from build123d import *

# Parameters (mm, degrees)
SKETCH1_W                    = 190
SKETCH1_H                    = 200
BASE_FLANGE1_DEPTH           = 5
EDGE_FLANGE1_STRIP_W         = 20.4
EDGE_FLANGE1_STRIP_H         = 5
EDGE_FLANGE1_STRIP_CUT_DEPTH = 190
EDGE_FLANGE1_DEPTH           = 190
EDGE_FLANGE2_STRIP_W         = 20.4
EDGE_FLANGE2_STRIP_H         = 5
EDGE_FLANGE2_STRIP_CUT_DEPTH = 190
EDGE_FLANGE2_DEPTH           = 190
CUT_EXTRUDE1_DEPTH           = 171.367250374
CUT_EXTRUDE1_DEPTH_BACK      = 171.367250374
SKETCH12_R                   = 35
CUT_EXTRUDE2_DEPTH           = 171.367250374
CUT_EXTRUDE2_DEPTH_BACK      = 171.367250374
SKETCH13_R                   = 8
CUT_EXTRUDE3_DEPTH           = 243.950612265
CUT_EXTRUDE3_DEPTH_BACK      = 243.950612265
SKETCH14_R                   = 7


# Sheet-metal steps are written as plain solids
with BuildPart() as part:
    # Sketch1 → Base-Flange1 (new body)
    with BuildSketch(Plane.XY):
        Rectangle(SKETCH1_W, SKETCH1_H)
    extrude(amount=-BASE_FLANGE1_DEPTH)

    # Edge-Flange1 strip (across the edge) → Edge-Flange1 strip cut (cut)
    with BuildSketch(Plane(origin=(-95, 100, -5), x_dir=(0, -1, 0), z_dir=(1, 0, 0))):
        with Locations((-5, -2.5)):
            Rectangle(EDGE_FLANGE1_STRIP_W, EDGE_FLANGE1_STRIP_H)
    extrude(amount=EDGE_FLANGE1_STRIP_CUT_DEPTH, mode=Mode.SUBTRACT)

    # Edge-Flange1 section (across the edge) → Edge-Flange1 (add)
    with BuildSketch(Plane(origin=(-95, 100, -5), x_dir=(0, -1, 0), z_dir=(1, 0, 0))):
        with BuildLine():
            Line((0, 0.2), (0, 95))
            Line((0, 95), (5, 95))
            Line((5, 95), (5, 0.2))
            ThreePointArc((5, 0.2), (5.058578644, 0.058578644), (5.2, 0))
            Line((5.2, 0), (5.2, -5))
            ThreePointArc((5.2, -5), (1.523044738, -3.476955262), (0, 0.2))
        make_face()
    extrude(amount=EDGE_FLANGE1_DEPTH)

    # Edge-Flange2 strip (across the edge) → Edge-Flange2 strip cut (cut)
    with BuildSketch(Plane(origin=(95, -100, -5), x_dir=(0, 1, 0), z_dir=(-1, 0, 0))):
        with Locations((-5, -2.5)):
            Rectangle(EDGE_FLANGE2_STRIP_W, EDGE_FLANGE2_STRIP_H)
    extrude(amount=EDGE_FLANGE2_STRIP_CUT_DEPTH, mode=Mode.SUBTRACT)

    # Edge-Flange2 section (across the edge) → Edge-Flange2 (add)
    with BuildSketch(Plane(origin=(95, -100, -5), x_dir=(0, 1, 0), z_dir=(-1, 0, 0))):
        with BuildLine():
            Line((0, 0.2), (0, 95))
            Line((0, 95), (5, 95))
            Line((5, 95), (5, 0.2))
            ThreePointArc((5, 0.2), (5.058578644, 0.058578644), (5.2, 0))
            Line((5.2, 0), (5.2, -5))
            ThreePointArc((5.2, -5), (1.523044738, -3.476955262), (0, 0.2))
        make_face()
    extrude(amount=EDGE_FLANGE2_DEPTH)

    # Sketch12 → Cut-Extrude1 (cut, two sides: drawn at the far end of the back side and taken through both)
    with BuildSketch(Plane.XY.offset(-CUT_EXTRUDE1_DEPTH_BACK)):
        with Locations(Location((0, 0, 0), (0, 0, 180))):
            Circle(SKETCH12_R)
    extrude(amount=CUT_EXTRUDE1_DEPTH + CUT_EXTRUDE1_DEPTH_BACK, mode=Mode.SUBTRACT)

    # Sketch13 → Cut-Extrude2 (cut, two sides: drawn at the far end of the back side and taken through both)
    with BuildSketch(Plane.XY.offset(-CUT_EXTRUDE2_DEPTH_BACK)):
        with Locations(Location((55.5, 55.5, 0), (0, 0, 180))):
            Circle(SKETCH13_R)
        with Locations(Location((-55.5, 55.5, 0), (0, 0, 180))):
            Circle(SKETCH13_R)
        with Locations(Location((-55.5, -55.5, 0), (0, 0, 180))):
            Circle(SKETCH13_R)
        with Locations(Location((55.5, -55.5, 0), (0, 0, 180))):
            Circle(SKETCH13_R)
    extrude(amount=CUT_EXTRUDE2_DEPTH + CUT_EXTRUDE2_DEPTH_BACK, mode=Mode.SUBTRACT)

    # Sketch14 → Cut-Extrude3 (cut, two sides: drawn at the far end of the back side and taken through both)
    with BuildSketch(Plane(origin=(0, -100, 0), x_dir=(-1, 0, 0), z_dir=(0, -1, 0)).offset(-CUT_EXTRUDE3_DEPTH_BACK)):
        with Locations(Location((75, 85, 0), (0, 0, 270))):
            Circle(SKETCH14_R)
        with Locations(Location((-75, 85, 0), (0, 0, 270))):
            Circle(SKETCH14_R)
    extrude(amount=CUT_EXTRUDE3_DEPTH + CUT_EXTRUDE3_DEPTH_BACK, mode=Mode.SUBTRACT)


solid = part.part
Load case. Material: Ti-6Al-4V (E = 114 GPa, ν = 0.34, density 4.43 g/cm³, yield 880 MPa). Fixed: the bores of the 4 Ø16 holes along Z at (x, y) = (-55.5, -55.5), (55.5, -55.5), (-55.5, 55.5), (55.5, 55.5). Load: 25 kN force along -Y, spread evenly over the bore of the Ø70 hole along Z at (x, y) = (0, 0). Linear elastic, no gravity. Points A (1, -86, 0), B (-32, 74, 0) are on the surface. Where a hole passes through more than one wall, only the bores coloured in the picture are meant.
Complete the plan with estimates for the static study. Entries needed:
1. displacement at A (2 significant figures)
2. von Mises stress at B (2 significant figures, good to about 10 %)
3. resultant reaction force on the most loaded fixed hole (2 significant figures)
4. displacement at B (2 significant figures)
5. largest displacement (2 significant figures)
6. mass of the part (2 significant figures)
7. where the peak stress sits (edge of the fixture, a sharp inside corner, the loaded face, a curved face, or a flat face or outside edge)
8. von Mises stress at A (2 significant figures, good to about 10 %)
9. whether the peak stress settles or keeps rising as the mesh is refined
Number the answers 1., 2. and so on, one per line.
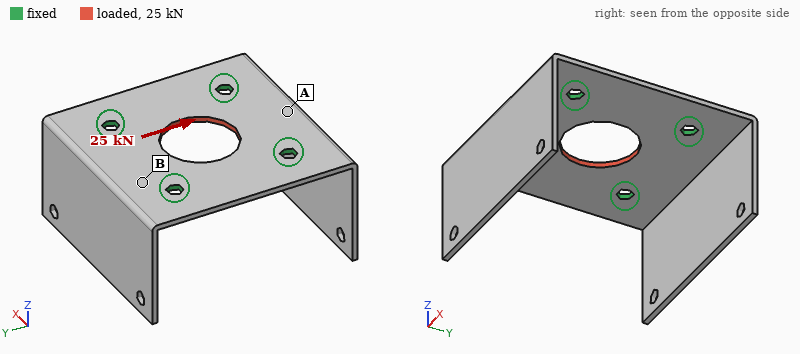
1. 11 µm
2. 18 MPa
3. 6.4 kN
4. 7.0 µm
5. 17 µm
6. 1.5 kg
7. edge of the fixture
8. 8.8 MPa
9. keeps rising
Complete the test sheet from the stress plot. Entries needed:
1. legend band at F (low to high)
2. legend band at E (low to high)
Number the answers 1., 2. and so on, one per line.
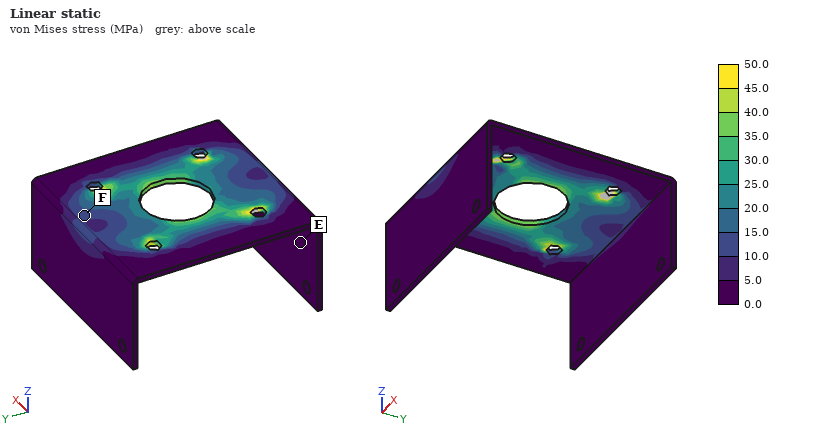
1. 10.0 to 15.0 MPa
2. 0.0 to 5.0 MPa
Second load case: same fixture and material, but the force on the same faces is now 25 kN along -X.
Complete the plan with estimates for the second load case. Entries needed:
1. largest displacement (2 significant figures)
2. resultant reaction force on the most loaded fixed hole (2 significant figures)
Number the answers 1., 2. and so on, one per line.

1. 18 µm
2. 6.5 kN
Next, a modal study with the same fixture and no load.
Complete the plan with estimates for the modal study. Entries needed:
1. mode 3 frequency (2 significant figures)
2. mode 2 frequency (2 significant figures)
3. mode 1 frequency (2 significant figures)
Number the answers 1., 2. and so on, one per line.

1. 510 Hz
2. 270 Hz
3. 270 Hz
